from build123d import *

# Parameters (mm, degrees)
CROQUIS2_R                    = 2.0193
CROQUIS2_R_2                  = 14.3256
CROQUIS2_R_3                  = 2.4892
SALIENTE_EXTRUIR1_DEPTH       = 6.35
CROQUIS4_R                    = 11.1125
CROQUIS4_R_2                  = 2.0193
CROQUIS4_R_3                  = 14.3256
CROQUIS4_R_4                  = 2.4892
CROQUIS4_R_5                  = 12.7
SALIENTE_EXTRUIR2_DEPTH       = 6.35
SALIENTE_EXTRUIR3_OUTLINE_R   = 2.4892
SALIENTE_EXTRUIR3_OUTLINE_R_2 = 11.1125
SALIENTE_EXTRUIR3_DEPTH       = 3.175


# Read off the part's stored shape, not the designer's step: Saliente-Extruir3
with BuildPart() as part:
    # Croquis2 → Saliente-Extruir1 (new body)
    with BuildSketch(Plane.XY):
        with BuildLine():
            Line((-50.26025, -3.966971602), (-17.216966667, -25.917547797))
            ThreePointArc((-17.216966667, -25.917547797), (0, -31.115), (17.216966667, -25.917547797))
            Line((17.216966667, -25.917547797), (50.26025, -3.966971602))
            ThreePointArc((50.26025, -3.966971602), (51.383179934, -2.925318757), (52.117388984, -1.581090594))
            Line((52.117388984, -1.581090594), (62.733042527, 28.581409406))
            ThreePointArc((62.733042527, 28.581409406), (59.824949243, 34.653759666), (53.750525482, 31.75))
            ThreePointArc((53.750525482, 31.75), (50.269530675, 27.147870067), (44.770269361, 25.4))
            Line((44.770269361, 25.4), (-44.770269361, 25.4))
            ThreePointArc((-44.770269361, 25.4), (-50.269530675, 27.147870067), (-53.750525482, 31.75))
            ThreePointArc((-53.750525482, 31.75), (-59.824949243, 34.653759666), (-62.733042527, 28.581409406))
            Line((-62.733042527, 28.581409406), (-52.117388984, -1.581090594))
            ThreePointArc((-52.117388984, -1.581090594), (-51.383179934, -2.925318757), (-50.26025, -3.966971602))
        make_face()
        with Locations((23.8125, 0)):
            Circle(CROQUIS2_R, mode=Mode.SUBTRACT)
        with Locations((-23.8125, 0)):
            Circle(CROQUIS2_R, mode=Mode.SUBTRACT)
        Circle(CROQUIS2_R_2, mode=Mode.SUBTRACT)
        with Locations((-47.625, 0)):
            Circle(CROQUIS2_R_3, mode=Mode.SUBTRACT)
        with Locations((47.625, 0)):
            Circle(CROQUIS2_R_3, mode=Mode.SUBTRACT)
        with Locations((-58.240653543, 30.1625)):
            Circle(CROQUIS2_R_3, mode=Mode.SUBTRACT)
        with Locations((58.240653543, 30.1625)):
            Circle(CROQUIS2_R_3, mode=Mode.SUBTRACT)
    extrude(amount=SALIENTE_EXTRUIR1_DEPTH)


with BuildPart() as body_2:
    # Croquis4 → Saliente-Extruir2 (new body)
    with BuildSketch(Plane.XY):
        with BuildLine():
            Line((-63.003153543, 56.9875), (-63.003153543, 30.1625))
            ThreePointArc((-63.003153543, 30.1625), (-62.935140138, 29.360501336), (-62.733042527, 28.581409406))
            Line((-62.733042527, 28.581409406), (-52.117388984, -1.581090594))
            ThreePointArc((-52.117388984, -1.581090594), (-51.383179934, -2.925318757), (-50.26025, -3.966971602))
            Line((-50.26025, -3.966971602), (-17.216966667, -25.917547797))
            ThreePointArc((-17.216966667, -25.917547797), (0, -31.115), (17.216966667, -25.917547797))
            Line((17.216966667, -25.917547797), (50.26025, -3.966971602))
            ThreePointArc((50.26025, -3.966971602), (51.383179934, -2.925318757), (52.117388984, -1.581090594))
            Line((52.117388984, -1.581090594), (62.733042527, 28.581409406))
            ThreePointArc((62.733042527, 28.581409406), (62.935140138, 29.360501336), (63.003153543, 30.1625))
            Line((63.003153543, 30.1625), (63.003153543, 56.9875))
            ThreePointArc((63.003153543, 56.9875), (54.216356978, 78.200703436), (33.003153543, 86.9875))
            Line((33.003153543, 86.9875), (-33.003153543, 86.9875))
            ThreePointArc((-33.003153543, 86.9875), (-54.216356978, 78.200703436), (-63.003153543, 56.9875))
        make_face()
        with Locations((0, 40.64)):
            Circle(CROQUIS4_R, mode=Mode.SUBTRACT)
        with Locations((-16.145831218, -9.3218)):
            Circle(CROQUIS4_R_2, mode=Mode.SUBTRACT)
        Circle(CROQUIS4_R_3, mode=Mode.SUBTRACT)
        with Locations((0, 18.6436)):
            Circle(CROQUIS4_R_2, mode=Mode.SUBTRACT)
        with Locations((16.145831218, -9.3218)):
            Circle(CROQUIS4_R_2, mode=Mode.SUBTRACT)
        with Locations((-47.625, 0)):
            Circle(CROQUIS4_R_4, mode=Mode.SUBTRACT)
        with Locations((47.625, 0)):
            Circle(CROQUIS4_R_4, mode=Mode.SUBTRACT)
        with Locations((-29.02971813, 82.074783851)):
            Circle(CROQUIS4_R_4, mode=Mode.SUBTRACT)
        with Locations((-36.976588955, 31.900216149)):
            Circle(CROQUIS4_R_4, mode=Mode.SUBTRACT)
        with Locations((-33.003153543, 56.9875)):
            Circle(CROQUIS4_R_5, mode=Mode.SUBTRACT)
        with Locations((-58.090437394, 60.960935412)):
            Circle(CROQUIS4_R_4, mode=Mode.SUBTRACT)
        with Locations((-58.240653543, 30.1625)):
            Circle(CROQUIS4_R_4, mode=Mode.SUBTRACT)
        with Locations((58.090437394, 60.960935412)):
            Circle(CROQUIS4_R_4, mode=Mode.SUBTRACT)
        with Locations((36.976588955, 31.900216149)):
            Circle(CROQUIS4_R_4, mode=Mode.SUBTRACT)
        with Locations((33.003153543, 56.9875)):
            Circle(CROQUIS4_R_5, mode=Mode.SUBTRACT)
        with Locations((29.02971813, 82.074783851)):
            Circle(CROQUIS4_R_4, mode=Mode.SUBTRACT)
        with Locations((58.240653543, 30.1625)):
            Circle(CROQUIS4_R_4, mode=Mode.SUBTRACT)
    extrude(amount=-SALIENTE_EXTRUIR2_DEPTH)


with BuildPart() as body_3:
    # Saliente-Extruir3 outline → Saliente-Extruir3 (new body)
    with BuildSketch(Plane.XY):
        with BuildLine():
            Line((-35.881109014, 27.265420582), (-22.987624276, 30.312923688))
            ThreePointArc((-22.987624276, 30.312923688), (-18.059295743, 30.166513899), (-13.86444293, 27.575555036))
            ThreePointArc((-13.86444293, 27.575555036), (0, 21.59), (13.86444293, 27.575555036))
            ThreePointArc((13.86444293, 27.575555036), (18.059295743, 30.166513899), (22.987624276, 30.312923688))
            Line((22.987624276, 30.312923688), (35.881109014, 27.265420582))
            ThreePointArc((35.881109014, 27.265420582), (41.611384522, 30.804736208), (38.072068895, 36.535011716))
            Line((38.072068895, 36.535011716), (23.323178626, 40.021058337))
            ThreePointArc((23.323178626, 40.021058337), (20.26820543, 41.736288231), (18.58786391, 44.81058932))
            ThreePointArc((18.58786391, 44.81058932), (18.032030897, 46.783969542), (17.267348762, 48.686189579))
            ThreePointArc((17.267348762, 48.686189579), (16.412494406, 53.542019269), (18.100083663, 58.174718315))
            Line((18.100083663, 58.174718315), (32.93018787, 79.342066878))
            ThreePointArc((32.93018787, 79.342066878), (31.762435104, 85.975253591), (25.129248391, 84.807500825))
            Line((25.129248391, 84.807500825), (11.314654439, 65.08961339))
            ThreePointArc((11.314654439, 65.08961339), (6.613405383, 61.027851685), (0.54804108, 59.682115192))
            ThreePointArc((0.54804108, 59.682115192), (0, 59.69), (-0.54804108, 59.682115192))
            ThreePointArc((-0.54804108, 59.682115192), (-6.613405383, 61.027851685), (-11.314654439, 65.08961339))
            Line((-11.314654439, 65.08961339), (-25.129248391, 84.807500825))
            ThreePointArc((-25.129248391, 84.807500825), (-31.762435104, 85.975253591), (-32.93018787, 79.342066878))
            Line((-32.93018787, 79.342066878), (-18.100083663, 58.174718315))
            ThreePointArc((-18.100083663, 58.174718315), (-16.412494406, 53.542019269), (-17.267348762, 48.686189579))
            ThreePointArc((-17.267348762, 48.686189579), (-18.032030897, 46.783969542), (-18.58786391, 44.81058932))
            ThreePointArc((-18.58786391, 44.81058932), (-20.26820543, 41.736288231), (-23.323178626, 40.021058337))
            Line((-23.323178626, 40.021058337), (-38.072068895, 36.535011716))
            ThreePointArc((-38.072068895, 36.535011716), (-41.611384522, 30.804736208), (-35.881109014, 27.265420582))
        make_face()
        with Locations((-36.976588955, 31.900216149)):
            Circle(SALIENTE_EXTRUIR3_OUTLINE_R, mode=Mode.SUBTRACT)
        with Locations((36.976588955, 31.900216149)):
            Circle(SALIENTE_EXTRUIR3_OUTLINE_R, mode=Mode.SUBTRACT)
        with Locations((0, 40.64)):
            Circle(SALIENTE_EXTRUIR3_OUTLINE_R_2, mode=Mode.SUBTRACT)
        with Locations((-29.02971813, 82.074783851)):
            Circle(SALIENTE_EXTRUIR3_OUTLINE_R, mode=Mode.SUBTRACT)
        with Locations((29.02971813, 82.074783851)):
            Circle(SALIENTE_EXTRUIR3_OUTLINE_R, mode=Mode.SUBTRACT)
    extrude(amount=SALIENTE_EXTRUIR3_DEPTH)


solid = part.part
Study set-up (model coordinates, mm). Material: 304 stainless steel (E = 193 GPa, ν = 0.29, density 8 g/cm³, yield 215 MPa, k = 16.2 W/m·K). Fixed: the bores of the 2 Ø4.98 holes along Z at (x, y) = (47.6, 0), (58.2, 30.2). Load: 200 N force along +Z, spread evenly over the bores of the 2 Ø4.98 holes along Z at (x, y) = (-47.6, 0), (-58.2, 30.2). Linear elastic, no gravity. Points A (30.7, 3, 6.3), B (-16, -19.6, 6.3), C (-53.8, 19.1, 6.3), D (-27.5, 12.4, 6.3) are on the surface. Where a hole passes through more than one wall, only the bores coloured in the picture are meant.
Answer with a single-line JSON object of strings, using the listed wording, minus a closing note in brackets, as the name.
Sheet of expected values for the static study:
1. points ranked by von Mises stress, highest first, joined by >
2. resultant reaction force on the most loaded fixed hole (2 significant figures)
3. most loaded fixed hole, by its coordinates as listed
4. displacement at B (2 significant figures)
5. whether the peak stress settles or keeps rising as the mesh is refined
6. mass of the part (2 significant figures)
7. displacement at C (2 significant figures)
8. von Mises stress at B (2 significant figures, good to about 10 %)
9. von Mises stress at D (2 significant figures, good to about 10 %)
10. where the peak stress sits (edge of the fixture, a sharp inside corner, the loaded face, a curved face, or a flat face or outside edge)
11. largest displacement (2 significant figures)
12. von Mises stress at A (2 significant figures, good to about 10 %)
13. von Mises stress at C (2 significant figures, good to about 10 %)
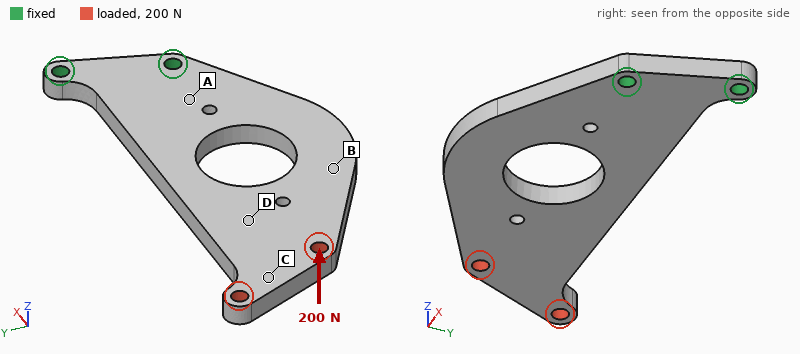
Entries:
{"points ranked by von Mises stress, highest first, joined by >": "A > B > D > C", "resultant reaction force on the most loaded fixed hole": "360 N", "most loaded fixed hole, by its coordinates as listed": "(47.6, 0)", "displacement at B": "0.23 mm", "whether the peak stress settles or keeps rising as the mesh is refined": "keeps rising", "mass of the part": "220 g", "displacement at C": "0.55 mm", "von Mises stress at B": "38 MPa", "von Mises stress at D": "20 MPa", "where the peak stress sits": "edge of the fixture", "largest displacement": "0.64 mm", "von Mises stress at A": "53 MPa", "von Mises stress at C": "12 MPa"}
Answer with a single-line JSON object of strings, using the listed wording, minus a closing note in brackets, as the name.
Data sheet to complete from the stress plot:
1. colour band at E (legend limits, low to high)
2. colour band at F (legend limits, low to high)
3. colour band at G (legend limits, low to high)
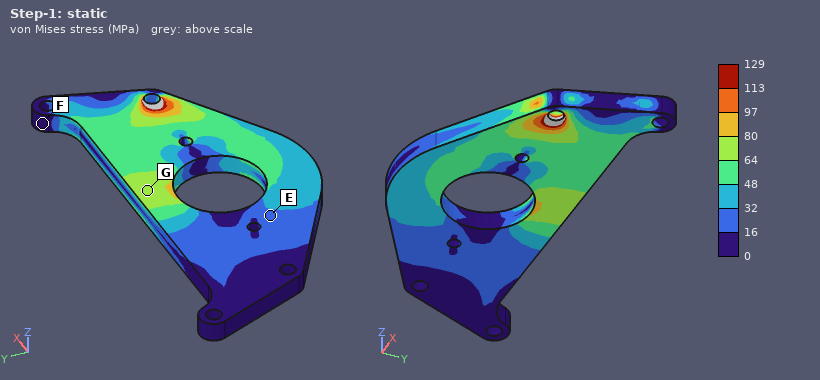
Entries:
{"colour band at E": "16 to 32 MPa", "colour band at F": "0 to 16 MPa", "colour band at G": "64 to 80 MPa"}
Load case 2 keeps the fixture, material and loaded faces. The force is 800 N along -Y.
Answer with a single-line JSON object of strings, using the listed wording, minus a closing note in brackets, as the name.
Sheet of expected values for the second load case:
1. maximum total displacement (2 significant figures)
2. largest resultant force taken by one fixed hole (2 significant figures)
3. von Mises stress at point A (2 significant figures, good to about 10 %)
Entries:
{"maximum total displacement": "0.10 mm", "largest resultant force taken by one fixed hole": "2.9 kN", "von Mises stress at point A": "26 MPa"}
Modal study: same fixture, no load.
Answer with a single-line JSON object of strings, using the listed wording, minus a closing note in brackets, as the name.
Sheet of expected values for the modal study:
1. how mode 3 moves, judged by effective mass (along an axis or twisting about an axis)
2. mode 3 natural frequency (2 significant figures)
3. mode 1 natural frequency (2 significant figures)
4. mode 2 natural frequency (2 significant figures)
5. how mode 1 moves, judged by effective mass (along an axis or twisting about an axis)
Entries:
{"how mode 3 moves, judged by effective mass": "along Y", "mode 3 natural frequency": "1800 Hz", "mode 1 natural frequency": "420 Hz", "mode 2 natural frequency": "1500 Hz", "how mode 1 moves, judged by effective mass": "along Z"}
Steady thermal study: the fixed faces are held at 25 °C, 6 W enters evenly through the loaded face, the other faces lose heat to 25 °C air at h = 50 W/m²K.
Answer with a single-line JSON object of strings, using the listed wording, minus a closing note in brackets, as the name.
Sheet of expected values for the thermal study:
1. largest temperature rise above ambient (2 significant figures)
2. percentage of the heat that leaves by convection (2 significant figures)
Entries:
{"largest temperature rise above ambient": "64 K", "percentage of the heat that leaves by convection": "97 %"}
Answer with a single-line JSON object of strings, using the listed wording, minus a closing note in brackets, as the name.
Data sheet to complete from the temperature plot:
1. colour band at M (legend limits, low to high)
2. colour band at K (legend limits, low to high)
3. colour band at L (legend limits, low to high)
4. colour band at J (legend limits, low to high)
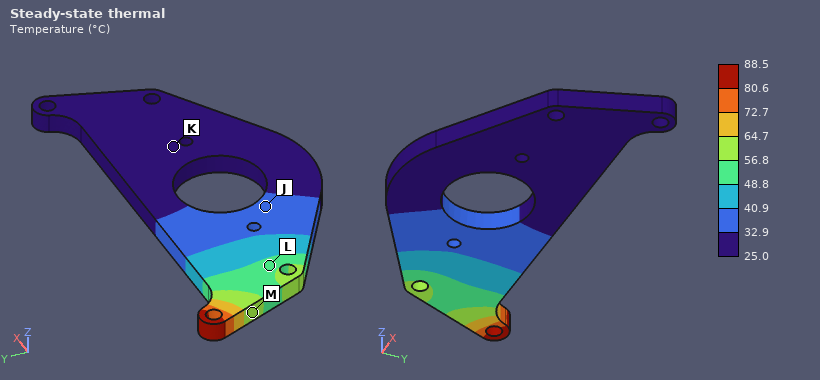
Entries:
{"colour band at M": "56.8 to 64.7 °C", "colour band at K": "25.0 to 32.9 °C", "colour band at L": "48.8 to 56.8 °C", "colour band at J": "32.9 to 40.9 °C"}
